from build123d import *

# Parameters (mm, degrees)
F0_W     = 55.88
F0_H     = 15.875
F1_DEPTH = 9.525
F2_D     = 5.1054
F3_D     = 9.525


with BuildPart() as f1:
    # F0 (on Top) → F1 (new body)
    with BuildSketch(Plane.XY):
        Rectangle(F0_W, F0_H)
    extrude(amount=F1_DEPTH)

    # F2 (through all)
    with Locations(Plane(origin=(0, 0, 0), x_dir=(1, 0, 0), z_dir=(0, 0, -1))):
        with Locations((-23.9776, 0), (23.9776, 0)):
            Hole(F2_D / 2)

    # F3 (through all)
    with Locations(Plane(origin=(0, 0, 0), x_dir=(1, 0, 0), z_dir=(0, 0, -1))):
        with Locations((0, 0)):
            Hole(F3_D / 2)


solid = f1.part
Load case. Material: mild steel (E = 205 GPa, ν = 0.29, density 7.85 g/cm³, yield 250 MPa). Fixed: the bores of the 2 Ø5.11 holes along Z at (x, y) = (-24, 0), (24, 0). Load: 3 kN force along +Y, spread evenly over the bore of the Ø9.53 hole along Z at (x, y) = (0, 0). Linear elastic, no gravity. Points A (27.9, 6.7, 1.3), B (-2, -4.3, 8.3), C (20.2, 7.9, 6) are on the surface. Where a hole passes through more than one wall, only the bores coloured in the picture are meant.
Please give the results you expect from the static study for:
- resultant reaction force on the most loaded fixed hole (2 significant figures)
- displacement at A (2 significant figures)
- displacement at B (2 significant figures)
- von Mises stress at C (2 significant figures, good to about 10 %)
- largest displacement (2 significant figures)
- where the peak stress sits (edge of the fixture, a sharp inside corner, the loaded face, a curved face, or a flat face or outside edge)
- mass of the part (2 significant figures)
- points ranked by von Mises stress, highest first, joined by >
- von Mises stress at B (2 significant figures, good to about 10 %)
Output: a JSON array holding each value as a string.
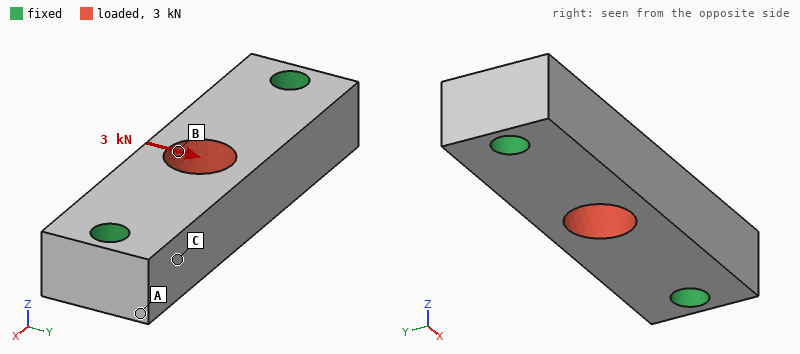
["1.5 kN", "1.4 µm", "7.5 µm", "20 MPa", "7.7 µm", "edge of the fixture", "58 g", "B > C > A", "34 MPa"]
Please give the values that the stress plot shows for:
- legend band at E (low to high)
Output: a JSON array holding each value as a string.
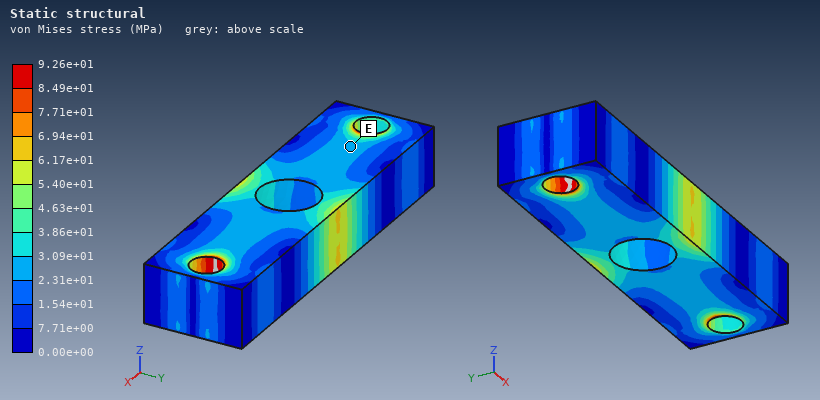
["2.31e+01 to 3.09e+01 MPa"]
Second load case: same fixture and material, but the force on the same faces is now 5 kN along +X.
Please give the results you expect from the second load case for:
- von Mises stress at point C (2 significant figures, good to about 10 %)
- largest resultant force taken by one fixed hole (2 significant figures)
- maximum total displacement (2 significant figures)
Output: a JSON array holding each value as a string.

["6.2 MPa", "2.5 kN", "2.1 µm"]
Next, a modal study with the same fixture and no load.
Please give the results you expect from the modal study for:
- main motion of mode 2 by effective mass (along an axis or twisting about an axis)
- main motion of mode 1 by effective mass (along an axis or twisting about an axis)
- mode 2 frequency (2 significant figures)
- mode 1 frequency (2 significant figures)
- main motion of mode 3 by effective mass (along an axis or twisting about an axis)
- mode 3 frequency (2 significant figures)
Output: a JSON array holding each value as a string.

["along Y", "along Z", "22 kHz", "19 kHz", "twisting about X", "29 kHz"]
